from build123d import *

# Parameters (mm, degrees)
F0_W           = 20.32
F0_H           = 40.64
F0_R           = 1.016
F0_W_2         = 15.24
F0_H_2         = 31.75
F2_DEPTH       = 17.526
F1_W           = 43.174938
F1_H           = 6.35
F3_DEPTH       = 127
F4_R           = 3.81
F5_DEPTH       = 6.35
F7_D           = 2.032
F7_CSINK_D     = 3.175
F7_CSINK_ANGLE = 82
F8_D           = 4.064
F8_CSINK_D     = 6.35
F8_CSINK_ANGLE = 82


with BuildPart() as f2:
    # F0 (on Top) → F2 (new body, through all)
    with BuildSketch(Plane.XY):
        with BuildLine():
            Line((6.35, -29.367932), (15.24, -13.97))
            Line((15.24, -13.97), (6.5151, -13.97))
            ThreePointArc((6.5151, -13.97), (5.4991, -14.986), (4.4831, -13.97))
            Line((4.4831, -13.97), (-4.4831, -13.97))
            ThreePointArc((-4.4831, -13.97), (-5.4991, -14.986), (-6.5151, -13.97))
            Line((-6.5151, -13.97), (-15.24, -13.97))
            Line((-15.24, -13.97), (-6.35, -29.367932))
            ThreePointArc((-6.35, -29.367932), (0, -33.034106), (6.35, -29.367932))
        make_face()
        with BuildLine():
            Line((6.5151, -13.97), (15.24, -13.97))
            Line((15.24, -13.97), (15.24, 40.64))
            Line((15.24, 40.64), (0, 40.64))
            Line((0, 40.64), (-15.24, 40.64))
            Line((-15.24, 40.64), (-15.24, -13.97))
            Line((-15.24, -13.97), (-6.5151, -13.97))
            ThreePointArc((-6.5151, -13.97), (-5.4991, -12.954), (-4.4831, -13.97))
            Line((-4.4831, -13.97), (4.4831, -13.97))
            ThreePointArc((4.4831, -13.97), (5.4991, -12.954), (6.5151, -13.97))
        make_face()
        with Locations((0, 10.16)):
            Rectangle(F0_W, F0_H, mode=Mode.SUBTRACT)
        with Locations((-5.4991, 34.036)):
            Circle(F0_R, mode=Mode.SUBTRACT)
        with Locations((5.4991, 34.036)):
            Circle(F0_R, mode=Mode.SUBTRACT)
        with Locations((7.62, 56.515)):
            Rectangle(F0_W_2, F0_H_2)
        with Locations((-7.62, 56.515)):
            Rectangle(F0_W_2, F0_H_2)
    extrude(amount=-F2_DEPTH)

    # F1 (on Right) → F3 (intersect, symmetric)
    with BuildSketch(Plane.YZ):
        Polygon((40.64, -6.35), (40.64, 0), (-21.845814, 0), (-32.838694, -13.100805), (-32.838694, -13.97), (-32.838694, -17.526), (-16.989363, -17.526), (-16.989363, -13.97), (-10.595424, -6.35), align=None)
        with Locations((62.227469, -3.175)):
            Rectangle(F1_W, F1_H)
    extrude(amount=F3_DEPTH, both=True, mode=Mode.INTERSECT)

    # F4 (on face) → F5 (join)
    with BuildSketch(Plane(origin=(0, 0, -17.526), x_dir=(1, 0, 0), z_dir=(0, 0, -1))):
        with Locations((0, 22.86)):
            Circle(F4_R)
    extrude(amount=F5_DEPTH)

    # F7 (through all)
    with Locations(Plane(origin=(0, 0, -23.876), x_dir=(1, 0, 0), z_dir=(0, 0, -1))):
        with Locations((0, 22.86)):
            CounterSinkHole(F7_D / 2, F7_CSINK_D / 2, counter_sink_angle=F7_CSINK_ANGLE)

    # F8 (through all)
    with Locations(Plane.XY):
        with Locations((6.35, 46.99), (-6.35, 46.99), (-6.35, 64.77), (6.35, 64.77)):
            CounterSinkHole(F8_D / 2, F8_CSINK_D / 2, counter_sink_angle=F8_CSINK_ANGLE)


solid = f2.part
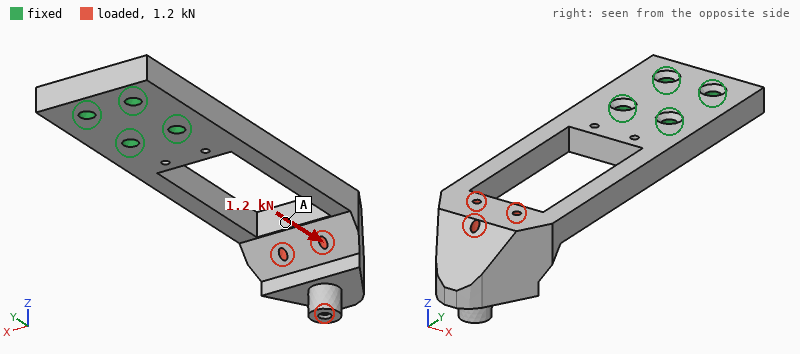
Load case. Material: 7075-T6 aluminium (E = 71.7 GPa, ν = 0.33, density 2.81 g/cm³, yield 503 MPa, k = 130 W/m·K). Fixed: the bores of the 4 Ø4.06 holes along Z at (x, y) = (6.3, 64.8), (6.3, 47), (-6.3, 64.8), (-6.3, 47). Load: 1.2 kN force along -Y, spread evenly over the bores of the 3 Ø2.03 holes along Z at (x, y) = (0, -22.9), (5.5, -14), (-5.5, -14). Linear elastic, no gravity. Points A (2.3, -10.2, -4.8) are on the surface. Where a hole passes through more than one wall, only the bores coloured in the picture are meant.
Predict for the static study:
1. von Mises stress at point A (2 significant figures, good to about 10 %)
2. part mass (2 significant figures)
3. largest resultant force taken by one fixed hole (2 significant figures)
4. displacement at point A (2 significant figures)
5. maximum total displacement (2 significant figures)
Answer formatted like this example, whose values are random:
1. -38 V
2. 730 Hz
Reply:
1. 16 MPa
2. 46 g
3. 540 N
4. 0.53 mm
5. 1.1 mm
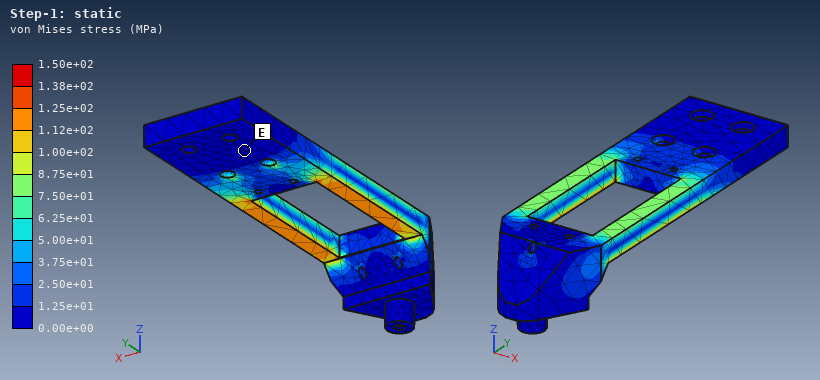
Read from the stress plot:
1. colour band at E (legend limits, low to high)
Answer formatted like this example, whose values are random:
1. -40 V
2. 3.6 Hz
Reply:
1. 0.00e+00 to 1.25e+01 MPa
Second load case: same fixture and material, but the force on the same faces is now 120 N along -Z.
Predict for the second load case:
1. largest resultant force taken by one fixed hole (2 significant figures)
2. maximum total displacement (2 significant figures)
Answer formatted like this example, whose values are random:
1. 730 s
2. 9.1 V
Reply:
1. 130 N
2. 0.72 mm
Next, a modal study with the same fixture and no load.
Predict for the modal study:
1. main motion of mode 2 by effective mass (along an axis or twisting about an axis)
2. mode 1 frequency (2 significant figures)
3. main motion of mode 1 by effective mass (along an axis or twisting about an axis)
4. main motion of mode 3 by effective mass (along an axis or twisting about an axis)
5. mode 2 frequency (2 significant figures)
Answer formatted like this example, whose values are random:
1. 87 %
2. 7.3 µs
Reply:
1. along X
2. 540 Hz
3. along Z
4. twisting about Y
5. 1100 Hz
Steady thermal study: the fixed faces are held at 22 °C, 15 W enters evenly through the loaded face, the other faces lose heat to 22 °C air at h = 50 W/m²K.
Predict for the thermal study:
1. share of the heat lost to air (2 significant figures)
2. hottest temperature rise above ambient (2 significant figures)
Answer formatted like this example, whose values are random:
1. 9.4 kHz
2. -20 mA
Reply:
1. 54 %
2. 54 K
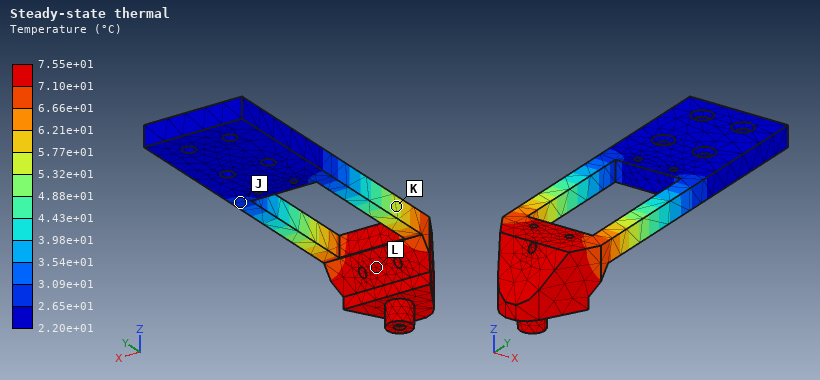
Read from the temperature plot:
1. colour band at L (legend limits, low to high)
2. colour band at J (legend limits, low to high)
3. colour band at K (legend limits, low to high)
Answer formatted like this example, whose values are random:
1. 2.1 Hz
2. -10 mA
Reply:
1. 7.10e+01 to 7.55e+01 °C
2. 2.65e+01 to 3.09e+01 °C
3. 5.32e+01 to 5.77e+01 °C
